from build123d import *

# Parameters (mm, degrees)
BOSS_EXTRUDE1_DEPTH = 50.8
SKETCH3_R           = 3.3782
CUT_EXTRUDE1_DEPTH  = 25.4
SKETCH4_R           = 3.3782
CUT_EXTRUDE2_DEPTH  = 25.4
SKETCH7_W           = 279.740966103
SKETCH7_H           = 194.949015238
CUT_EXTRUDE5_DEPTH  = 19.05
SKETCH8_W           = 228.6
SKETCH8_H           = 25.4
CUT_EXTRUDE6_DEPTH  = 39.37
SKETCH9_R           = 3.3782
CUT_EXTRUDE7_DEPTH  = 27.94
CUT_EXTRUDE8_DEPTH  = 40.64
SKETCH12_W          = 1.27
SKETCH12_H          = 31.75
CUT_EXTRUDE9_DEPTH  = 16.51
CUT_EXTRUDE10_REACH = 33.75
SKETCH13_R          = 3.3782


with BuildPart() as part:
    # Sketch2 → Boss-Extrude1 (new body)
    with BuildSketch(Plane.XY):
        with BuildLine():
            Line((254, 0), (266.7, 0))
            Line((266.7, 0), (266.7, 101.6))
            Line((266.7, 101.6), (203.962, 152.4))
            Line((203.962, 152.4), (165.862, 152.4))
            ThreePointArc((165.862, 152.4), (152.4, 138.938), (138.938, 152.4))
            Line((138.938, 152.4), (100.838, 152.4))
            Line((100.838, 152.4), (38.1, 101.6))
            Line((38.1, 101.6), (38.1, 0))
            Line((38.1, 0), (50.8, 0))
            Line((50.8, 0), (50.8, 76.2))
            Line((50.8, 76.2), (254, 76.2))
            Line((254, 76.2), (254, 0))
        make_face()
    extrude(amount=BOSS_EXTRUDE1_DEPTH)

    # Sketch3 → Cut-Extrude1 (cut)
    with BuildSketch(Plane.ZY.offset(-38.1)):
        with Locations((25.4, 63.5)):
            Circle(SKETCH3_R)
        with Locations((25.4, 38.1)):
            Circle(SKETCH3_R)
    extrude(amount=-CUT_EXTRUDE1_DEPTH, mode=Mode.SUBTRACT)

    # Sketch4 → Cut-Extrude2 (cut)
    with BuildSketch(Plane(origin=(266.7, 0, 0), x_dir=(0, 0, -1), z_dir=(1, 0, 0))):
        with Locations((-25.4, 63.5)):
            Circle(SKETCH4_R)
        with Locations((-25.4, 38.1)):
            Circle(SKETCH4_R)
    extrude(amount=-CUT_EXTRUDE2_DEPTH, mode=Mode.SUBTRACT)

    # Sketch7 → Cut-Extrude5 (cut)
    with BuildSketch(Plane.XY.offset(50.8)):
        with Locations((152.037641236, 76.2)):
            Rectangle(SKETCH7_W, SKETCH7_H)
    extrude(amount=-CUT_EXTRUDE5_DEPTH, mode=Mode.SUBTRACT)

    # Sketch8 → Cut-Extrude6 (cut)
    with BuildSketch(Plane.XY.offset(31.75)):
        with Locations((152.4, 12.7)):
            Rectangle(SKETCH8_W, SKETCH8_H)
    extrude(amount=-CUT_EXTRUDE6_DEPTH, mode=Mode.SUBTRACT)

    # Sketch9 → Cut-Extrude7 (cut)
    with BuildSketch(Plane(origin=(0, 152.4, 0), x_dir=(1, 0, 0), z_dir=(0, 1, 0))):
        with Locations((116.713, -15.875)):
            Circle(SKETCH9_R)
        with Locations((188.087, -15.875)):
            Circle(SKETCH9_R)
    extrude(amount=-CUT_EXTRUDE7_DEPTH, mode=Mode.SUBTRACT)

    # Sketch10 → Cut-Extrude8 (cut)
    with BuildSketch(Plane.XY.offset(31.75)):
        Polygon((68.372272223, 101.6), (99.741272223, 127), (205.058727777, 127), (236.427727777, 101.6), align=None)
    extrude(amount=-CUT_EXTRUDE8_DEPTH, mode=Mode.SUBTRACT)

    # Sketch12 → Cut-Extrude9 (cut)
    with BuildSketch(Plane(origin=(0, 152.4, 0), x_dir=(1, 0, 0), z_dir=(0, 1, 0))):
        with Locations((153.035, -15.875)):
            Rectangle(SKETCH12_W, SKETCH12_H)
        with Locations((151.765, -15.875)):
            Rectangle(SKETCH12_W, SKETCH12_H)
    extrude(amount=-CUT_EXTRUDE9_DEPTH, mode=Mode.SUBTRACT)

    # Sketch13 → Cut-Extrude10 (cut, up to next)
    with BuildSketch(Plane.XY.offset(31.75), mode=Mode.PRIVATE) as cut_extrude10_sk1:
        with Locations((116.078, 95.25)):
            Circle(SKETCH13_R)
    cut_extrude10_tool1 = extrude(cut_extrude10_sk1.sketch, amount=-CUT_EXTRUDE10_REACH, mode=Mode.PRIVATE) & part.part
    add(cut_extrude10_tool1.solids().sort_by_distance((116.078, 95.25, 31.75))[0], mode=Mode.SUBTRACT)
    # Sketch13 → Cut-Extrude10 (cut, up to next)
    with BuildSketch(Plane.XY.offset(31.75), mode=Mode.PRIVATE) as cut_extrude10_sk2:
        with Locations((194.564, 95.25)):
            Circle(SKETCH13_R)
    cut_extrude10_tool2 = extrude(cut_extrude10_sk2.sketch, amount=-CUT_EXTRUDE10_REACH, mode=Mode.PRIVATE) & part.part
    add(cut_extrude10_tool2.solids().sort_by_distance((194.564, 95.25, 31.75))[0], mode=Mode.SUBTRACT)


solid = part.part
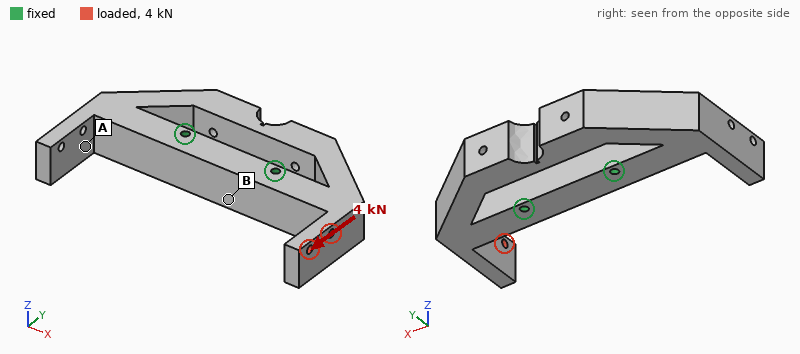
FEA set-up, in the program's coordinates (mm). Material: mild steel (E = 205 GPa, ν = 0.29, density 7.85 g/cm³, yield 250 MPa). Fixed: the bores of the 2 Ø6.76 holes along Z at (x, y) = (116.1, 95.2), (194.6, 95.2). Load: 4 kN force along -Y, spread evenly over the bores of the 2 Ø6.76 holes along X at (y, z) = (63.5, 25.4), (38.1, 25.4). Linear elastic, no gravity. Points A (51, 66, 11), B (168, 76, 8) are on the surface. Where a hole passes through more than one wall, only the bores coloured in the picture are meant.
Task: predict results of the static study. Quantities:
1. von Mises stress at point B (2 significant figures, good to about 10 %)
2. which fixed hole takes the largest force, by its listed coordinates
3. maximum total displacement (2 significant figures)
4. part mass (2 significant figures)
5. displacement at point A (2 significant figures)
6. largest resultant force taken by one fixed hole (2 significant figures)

17 MPa
(194.6, 95.2)
78 µm
2.9 kg
15 µm
6.3 kN
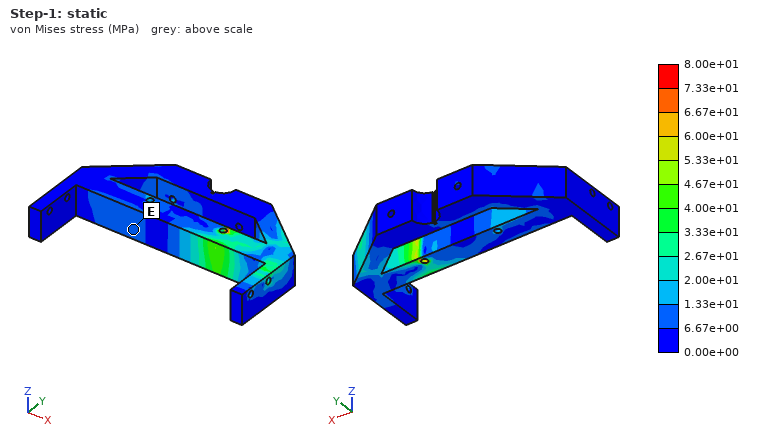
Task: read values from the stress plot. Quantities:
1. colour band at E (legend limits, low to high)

6.67e+00 to 1.33e+01 MPa
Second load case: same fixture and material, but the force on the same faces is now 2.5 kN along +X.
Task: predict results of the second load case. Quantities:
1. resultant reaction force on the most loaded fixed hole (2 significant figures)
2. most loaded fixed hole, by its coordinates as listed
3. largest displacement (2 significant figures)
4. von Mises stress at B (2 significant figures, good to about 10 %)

2.4 kN
(194.6, 95.2)
0.10 mm
6.1 MPa
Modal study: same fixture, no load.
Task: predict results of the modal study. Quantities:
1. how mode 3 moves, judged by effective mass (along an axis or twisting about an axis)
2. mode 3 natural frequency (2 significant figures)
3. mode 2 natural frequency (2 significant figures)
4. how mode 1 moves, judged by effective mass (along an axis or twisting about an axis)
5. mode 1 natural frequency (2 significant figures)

along Y
1800 Hz
1500 Hz
along Z
1400 Hz
